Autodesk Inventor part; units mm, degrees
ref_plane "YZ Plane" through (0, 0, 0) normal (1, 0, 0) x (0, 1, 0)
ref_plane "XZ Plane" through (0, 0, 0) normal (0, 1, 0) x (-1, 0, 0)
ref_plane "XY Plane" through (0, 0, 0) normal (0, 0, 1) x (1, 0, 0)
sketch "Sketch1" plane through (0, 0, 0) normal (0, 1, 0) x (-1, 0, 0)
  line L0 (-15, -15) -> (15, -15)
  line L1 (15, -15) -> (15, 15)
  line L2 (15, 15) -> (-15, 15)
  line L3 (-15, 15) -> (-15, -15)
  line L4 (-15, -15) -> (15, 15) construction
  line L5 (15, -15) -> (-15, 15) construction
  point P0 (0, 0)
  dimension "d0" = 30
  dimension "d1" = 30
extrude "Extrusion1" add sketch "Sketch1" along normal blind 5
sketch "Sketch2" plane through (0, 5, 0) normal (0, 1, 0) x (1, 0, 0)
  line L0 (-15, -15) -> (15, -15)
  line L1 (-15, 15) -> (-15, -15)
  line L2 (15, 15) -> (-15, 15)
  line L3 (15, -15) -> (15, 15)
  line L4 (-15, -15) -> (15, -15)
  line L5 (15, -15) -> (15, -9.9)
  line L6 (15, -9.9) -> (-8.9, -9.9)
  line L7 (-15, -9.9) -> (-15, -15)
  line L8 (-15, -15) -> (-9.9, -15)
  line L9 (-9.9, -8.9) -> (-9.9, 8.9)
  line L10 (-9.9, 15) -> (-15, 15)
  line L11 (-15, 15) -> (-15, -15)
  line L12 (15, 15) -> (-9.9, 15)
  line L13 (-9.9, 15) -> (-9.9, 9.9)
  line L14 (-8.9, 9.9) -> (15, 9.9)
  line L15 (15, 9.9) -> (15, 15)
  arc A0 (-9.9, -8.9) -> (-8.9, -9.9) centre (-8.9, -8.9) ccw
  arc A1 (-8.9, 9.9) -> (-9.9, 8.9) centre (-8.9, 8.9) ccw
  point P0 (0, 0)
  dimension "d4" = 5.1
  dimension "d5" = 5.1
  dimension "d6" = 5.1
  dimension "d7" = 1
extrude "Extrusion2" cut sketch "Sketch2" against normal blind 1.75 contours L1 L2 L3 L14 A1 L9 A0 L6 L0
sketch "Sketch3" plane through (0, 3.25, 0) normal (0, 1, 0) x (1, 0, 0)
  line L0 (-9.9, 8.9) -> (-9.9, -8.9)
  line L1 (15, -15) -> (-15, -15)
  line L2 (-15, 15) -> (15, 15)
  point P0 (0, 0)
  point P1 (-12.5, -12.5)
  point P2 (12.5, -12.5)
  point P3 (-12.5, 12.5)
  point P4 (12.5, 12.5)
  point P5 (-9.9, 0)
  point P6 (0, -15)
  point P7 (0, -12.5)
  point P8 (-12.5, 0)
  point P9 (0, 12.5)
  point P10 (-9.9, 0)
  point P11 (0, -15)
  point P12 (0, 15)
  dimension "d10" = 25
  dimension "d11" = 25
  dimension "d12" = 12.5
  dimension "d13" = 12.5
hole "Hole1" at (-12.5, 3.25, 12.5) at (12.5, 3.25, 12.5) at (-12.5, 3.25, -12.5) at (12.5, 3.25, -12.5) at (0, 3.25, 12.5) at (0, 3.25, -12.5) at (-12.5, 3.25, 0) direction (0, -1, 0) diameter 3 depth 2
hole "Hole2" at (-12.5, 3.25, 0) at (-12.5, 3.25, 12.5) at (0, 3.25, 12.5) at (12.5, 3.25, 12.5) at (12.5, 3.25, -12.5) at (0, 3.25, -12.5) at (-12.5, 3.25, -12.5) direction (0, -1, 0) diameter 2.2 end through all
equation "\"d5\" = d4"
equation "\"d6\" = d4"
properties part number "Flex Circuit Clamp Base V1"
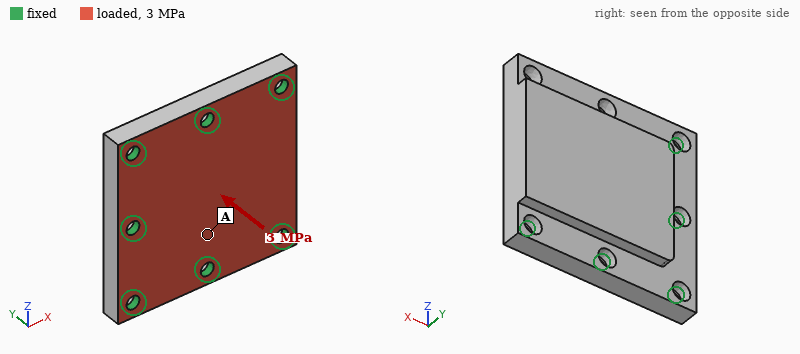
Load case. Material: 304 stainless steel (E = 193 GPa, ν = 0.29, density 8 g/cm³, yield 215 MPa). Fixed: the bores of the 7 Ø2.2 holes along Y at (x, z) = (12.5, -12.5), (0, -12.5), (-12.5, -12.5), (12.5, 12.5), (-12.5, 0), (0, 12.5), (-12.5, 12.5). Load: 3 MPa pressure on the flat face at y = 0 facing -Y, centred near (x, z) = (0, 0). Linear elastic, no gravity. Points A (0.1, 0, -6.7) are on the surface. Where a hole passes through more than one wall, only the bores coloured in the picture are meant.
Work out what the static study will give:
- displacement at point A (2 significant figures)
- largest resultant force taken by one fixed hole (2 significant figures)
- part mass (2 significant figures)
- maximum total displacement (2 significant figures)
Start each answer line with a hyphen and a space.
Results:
- 2.8 µm
- 550 N
- 29 g
- 5.0 µm
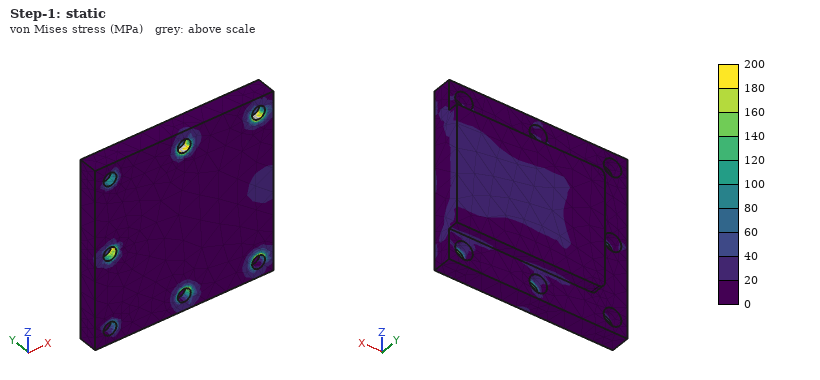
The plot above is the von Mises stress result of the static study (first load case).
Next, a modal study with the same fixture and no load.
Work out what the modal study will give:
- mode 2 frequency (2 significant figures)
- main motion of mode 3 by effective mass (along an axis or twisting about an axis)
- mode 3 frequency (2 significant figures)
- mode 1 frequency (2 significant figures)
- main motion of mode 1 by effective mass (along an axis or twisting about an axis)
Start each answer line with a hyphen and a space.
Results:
- 37 kHz
- along Z
- 48 kHz
- 24 kHz
- along Y
